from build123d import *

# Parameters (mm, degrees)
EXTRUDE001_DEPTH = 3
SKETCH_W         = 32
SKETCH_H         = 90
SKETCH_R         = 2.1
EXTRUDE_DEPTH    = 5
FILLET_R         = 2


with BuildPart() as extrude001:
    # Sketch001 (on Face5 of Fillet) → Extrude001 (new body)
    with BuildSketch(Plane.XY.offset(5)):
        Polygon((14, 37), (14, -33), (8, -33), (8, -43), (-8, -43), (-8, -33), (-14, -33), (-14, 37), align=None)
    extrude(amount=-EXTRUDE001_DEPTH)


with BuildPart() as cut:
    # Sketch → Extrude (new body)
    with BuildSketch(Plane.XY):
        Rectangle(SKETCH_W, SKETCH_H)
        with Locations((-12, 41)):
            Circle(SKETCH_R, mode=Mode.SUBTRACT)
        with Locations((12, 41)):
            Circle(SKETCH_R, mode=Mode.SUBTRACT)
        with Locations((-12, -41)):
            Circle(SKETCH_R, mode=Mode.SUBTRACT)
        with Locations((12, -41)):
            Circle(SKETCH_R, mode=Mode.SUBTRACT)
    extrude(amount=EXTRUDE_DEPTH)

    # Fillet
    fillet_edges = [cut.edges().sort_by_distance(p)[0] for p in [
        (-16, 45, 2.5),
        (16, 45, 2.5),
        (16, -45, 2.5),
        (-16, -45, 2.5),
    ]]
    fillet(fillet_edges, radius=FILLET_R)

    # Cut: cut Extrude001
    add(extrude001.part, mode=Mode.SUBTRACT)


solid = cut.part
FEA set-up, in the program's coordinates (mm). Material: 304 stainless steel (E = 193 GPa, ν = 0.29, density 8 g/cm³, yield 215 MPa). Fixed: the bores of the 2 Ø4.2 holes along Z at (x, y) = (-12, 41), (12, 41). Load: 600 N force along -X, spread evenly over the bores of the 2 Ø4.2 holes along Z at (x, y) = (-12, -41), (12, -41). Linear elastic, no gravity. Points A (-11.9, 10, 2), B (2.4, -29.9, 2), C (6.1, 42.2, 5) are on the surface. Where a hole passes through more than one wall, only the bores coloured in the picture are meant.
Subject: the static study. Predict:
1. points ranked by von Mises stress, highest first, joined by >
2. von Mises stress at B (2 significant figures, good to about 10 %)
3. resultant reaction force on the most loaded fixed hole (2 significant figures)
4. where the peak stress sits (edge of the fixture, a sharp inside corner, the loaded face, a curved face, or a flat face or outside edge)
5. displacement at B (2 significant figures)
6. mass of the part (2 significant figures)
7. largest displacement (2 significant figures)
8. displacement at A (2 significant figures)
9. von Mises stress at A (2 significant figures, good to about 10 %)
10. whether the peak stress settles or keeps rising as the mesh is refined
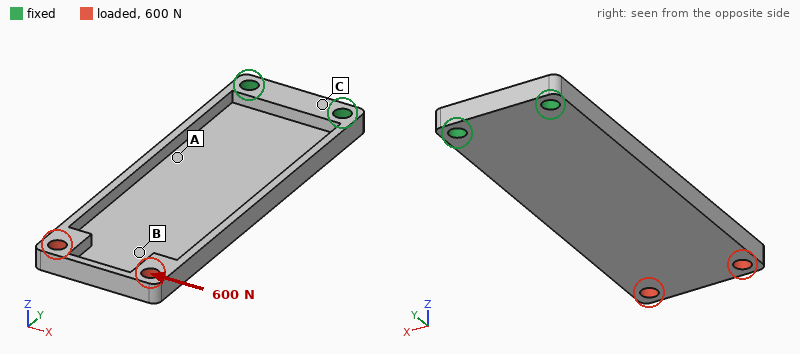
A > B > C
46 MPa
1.9 kN
edge of the fixture
0.080 mm
62 g
0.19 mm
0.039 mm
65 MPa
keeps rising
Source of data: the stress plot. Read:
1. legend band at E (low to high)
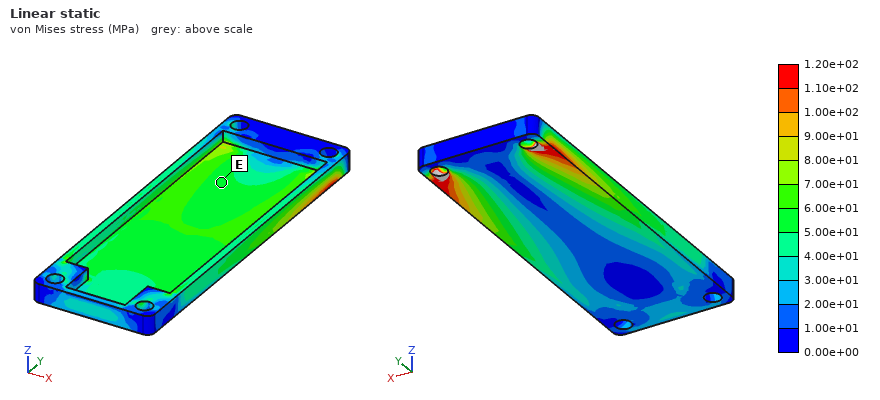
5.00e+01 to 6.00e+01 MPa
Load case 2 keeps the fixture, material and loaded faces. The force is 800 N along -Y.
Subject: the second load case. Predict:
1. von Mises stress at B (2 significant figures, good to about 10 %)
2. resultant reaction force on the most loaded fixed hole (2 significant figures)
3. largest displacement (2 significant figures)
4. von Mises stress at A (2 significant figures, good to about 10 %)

15 MPa
400 N
0.17 mm
16 MPa
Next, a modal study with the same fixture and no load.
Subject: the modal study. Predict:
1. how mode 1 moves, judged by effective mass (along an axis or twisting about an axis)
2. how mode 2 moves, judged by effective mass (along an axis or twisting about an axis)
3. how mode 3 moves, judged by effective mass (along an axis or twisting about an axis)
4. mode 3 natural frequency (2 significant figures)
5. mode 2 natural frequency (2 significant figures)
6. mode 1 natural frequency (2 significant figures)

along Z
twisting about Y
along Z
2400 Hz
1300 Hz
390 Hz
